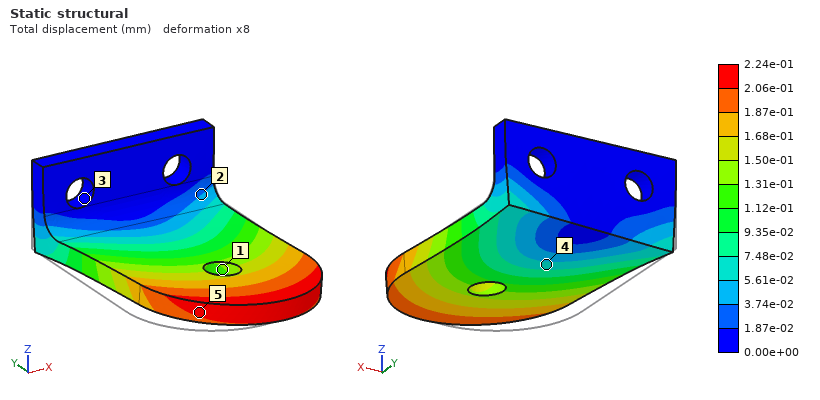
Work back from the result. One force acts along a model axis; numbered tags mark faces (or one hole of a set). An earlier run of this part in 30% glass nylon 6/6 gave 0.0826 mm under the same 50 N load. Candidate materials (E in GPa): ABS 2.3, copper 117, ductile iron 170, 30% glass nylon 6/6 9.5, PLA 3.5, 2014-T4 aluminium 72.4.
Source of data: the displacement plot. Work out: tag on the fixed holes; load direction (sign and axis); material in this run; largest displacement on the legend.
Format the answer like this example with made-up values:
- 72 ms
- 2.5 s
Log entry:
- 3
- +X
- PLA
- 2.24e-01 mm
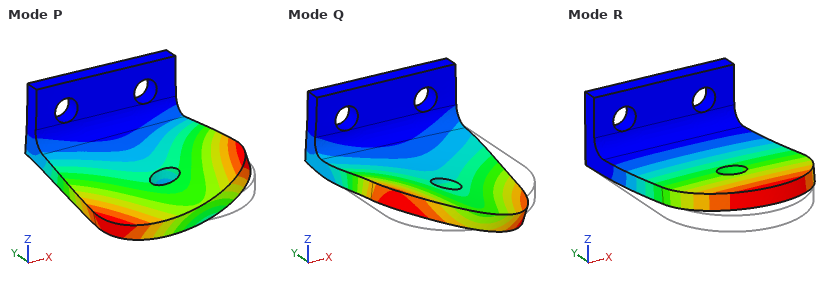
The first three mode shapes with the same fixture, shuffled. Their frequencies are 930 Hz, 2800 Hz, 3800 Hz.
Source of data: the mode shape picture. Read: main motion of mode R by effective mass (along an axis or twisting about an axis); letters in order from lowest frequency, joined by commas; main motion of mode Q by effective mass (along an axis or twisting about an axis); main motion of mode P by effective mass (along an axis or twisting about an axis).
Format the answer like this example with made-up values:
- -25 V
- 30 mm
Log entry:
- along Z
- R, P, Q
- along X
- along X
